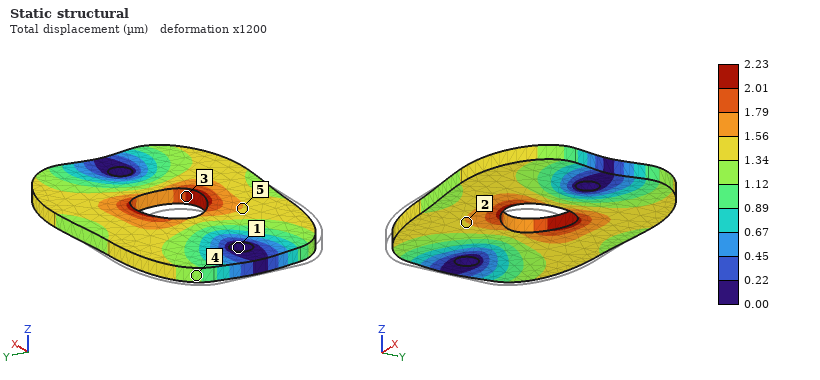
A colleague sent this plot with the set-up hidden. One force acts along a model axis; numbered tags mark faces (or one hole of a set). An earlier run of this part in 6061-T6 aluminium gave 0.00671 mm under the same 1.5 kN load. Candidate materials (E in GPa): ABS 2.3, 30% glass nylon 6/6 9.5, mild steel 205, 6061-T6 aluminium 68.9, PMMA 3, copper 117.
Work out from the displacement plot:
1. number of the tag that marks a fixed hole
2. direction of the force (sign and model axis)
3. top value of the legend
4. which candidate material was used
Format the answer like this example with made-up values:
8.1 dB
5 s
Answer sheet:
1
+X
2.23 µm
mild steel
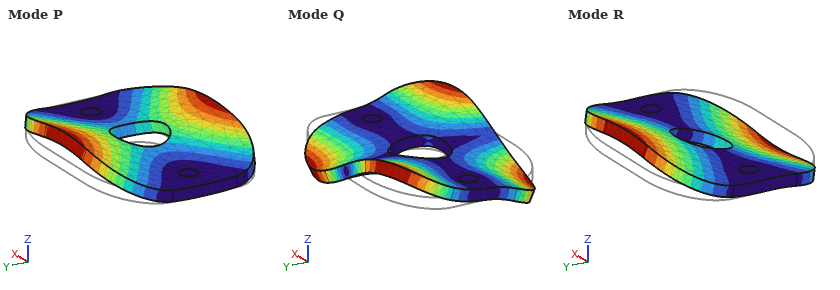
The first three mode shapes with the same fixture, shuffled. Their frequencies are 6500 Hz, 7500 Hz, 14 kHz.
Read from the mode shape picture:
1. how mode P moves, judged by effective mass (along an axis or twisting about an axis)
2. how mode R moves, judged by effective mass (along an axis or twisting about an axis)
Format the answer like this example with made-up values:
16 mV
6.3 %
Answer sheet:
along Z
twisting about X
